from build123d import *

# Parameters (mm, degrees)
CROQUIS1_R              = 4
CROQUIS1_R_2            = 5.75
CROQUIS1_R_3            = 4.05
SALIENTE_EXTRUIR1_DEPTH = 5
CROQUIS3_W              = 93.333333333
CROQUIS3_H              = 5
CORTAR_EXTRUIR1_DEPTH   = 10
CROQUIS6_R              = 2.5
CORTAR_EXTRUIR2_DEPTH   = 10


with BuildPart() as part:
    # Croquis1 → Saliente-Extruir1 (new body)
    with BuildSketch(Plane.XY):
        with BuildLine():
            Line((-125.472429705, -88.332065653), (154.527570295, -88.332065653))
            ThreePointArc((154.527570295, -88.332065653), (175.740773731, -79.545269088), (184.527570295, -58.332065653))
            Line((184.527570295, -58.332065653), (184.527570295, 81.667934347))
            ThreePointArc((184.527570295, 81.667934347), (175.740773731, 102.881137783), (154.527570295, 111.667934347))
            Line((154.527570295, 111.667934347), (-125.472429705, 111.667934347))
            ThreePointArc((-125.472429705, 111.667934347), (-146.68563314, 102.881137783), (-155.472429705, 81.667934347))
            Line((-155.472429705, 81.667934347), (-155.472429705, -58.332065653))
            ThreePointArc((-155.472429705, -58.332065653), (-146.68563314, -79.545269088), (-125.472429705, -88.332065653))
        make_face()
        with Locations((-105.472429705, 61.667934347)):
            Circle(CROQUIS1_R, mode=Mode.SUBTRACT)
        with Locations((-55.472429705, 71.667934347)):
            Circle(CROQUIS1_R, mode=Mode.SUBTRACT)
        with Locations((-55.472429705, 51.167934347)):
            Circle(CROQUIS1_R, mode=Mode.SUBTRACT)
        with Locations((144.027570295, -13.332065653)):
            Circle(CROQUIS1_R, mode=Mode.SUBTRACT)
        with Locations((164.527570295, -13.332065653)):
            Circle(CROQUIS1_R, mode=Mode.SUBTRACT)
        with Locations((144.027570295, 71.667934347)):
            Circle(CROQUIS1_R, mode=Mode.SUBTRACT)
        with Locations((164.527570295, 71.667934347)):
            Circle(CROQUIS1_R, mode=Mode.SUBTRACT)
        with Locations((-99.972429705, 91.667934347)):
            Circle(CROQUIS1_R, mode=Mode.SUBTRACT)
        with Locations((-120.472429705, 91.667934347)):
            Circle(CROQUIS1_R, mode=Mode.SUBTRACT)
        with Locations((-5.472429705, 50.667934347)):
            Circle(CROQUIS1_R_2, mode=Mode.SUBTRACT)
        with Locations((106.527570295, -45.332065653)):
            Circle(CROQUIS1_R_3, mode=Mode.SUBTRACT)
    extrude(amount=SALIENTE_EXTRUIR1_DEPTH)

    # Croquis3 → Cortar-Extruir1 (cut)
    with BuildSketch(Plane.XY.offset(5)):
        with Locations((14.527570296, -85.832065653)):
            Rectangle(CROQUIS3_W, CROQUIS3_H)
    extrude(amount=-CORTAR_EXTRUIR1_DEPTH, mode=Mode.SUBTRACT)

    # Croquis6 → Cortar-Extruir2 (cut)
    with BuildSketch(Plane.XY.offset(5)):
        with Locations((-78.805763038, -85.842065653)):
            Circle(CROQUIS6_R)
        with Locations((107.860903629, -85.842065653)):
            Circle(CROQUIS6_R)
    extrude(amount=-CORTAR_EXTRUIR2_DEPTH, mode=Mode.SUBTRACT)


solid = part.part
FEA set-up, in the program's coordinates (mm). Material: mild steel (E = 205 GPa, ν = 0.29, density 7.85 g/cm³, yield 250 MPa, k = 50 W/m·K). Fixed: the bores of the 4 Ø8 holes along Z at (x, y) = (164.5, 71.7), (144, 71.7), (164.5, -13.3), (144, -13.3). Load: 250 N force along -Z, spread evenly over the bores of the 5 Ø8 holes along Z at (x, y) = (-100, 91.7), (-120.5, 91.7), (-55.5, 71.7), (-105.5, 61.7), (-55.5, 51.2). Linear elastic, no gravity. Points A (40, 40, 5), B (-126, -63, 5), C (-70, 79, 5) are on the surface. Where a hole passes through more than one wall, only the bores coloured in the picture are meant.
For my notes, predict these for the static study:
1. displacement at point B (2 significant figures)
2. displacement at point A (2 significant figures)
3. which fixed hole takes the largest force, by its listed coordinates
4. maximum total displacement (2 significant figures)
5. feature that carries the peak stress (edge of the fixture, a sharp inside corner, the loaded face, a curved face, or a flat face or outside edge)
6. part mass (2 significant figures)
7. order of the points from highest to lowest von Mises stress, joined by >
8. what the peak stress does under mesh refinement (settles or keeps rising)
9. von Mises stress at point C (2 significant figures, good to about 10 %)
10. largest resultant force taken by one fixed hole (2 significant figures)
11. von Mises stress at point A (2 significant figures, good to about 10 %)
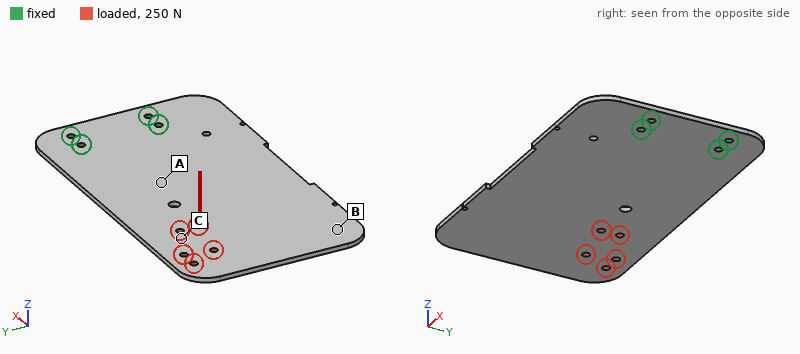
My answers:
2.8 mm
0.72 mm
(144, 71.7)
4.0 mm
edge of the fixture
2.6 kg
A > C > B
keeps rising
17 MPa
810 N
39 MPa
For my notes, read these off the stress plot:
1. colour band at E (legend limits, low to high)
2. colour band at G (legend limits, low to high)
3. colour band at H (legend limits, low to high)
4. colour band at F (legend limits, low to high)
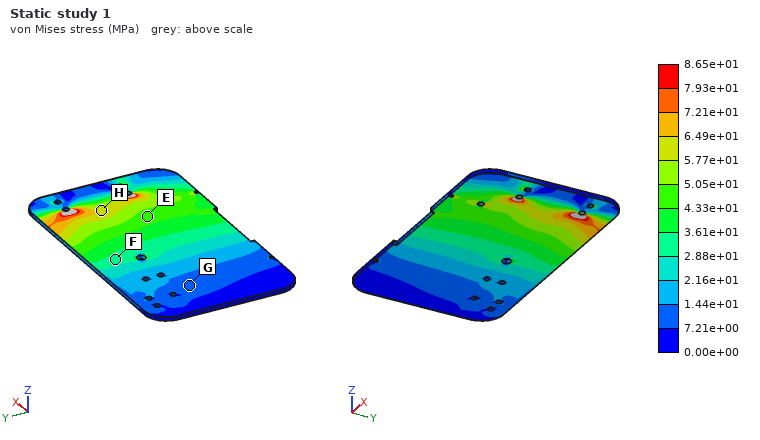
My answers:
4.33e+01 to 5.05e+01 MPa
7.21e+00 to 1.44e+01 MPa
5.77e+01 to 6.49e+01 MPa
2.88e+01 to 3.61e+01 MPa
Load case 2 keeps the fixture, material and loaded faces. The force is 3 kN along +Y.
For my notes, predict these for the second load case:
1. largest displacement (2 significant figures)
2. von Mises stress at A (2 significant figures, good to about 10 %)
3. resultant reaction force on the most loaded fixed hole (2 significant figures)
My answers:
73 µm
9.4 MPa
5.6 kN
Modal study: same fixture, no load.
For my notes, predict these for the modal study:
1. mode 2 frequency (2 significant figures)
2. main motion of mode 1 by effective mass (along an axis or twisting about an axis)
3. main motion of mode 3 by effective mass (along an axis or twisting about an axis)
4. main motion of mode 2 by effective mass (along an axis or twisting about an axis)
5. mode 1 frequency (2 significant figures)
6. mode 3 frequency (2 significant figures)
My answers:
150 Hz
along Z
along Z
twisting about X
46 Hz
280 Hz
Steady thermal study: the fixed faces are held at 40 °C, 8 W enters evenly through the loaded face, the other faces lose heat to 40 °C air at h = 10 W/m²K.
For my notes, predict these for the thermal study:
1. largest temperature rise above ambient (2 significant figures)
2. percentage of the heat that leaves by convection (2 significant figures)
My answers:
18 K
86 %
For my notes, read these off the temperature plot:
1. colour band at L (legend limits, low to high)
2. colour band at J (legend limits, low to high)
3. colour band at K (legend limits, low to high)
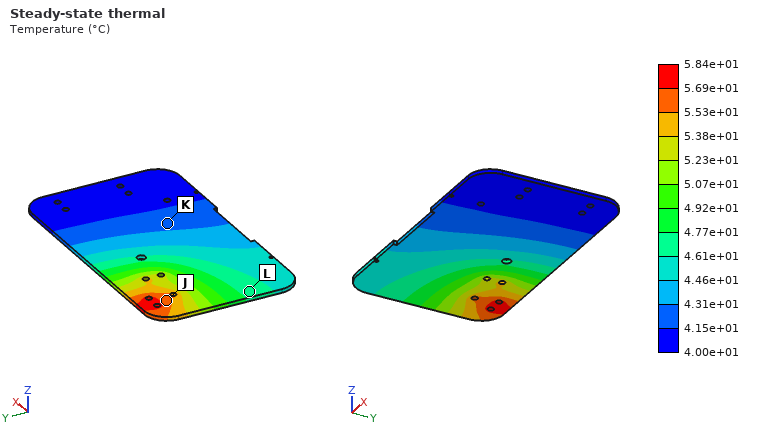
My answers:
4.61e+01 to 4.77e+01 °C
5.53e+01 to 5.69e+01 °C
4.15e+01 to 4.31e+01 °C
